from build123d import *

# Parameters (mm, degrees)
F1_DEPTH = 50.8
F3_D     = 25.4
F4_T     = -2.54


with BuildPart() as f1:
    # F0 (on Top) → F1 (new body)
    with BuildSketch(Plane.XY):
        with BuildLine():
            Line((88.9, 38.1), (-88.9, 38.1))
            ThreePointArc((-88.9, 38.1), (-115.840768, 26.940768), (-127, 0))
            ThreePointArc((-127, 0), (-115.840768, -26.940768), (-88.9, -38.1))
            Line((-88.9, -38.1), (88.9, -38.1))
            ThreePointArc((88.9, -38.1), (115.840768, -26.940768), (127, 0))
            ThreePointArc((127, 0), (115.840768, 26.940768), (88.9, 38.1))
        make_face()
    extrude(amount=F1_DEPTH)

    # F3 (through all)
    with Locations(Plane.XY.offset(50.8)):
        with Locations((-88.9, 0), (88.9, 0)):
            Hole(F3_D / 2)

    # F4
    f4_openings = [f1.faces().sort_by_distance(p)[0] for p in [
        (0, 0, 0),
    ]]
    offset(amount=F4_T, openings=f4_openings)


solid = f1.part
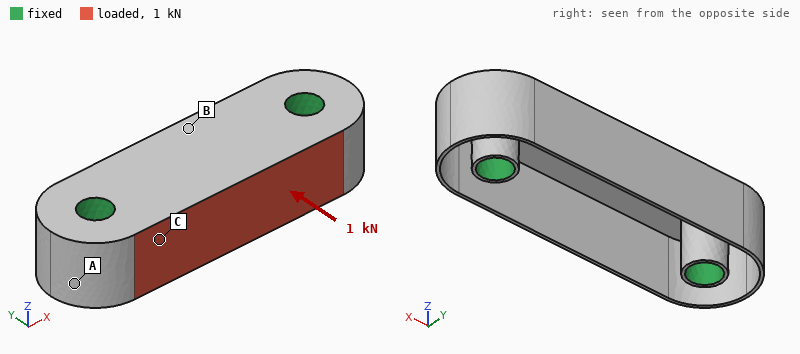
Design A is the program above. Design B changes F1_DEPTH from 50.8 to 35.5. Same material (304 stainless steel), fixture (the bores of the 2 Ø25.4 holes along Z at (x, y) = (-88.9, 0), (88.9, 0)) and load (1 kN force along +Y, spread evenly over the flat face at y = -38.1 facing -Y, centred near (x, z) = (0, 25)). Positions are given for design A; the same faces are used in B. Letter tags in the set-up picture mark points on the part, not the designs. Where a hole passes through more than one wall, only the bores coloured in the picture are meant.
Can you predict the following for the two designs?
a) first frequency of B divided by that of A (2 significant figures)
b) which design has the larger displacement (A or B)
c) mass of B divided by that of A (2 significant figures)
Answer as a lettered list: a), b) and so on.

a) 1.4
b) A
c) 0.78
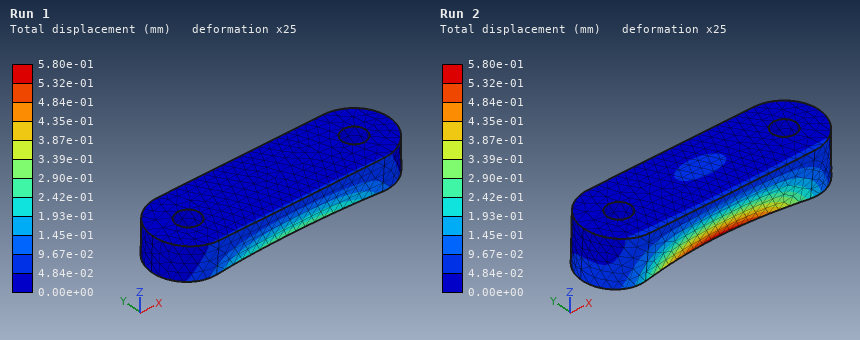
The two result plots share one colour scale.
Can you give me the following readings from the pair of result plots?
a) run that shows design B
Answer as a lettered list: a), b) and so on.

a) Run 1
